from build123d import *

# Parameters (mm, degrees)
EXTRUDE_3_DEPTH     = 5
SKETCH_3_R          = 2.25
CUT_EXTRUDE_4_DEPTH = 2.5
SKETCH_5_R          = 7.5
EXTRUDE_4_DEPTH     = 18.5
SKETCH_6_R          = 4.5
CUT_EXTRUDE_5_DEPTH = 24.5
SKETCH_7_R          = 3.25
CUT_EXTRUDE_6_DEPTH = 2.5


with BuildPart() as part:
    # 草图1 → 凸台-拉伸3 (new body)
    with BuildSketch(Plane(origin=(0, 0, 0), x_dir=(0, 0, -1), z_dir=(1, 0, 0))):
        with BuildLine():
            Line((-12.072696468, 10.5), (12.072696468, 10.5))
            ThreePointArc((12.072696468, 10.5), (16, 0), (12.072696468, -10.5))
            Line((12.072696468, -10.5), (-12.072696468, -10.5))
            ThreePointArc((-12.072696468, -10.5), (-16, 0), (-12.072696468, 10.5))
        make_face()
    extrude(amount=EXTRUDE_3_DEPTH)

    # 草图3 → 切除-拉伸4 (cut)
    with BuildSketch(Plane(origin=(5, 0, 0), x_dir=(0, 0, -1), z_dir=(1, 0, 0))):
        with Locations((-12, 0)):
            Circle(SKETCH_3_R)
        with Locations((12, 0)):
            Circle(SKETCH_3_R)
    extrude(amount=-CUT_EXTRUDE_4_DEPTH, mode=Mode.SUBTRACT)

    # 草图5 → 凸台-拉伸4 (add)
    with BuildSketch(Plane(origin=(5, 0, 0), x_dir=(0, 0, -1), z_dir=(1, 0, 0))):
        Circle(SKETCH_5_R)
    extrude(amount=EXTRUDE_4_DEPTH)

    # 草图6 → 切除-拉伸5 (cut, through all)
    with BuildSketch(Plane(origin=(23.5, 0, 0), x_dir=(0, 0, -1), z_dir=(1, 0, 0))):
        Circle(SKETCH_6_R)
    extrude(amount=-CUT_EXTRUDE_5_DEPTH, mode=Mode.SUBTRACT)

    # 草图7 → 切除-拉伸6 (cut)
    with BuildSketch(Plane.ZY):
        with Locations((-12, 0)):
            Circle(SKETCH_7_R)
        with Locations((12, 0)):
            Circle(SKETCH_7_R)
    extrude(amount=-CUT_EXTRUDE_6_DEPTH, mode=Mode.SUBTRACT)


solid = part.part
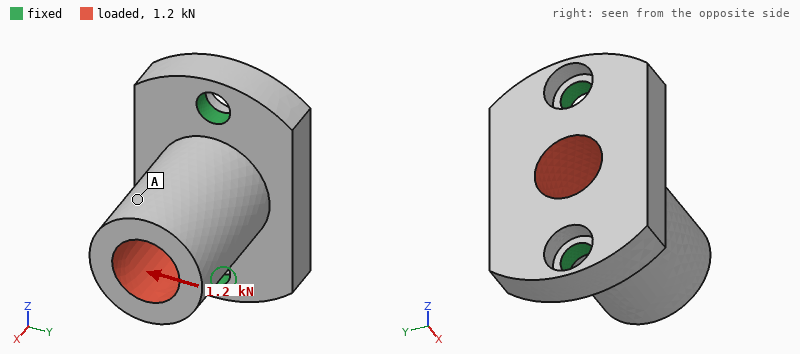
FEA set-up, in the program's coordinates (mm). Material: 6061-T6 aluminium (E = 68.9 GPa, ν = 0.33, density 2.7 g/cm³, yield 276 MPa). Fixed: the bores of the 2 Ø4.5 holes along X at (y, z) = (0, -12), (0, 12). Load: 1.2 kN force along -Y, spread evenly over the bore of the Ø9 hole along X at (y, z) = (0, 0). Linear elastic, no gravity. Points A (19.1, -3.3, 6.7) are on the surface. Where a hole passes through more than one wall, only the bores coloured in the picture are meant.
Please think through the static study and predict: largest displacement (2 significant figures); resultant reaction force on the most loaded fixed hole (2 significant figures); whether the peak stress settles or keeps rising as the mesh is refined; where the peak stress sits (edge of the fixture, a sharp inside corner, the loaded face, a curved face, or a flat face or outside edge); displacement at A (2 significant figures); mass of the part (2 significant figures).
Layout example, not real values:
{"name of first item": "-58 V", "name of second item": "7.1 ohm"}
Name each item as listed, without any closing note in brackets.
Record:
{"largest displacement": "95 µm", "resultant reaction force on the most loaded fixed hole": "600 N", "whether the peak stress settles or keeps rising as the mesh is refined": "keeps rising", "where the peak stress sits": "edge of the fixture", "displacement at A": "71 µm", "mass of the part": "12 g"}
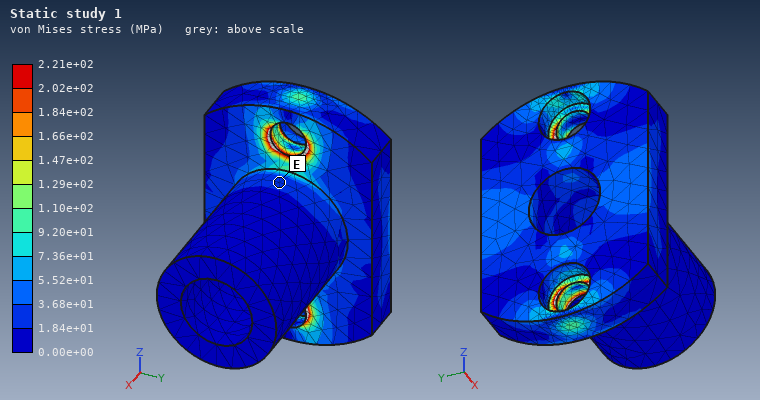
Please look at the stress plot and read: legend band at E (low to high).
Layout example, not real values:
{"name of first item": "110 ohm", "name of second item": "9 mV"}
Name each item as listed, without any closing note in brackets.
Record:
{"legend band at E": "1.84e+01 to 3.68e+01 MPa"}
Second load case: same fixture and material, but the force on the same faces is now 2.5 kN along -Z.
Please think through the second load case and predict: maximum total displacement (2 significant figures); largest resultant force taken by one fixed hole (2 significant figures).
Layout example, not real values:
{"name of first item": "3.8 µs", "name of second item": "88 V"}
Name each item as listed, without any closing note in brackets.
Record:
{"maximum total displacement": "49 µm", "largest resultant force taken by one fixed hole": "1.6 kN"}
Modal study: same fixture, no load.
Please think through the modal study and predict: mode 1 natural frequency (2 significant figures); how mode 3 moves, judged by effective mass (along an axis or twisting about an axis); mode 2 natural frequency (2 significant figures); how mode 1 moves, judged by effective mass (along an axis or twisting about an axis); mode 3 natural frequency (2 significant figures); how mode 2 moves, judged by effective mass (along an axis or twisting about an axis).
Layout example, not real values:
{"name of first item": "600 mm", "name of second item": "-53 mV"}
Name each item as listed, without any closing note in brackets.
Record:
{"mode 1 natural frequency": "7200 Hz", "how mode 3 moves, judged by effective mass": "along X", "mode 2 natural frequency": "16 kHz", "how mode 1 moves, judged by effective mass": "along Y", "mode 3 natural frequency": "20 kHz", "how mode 2 moves, judged by effective mass": "along Z"}
